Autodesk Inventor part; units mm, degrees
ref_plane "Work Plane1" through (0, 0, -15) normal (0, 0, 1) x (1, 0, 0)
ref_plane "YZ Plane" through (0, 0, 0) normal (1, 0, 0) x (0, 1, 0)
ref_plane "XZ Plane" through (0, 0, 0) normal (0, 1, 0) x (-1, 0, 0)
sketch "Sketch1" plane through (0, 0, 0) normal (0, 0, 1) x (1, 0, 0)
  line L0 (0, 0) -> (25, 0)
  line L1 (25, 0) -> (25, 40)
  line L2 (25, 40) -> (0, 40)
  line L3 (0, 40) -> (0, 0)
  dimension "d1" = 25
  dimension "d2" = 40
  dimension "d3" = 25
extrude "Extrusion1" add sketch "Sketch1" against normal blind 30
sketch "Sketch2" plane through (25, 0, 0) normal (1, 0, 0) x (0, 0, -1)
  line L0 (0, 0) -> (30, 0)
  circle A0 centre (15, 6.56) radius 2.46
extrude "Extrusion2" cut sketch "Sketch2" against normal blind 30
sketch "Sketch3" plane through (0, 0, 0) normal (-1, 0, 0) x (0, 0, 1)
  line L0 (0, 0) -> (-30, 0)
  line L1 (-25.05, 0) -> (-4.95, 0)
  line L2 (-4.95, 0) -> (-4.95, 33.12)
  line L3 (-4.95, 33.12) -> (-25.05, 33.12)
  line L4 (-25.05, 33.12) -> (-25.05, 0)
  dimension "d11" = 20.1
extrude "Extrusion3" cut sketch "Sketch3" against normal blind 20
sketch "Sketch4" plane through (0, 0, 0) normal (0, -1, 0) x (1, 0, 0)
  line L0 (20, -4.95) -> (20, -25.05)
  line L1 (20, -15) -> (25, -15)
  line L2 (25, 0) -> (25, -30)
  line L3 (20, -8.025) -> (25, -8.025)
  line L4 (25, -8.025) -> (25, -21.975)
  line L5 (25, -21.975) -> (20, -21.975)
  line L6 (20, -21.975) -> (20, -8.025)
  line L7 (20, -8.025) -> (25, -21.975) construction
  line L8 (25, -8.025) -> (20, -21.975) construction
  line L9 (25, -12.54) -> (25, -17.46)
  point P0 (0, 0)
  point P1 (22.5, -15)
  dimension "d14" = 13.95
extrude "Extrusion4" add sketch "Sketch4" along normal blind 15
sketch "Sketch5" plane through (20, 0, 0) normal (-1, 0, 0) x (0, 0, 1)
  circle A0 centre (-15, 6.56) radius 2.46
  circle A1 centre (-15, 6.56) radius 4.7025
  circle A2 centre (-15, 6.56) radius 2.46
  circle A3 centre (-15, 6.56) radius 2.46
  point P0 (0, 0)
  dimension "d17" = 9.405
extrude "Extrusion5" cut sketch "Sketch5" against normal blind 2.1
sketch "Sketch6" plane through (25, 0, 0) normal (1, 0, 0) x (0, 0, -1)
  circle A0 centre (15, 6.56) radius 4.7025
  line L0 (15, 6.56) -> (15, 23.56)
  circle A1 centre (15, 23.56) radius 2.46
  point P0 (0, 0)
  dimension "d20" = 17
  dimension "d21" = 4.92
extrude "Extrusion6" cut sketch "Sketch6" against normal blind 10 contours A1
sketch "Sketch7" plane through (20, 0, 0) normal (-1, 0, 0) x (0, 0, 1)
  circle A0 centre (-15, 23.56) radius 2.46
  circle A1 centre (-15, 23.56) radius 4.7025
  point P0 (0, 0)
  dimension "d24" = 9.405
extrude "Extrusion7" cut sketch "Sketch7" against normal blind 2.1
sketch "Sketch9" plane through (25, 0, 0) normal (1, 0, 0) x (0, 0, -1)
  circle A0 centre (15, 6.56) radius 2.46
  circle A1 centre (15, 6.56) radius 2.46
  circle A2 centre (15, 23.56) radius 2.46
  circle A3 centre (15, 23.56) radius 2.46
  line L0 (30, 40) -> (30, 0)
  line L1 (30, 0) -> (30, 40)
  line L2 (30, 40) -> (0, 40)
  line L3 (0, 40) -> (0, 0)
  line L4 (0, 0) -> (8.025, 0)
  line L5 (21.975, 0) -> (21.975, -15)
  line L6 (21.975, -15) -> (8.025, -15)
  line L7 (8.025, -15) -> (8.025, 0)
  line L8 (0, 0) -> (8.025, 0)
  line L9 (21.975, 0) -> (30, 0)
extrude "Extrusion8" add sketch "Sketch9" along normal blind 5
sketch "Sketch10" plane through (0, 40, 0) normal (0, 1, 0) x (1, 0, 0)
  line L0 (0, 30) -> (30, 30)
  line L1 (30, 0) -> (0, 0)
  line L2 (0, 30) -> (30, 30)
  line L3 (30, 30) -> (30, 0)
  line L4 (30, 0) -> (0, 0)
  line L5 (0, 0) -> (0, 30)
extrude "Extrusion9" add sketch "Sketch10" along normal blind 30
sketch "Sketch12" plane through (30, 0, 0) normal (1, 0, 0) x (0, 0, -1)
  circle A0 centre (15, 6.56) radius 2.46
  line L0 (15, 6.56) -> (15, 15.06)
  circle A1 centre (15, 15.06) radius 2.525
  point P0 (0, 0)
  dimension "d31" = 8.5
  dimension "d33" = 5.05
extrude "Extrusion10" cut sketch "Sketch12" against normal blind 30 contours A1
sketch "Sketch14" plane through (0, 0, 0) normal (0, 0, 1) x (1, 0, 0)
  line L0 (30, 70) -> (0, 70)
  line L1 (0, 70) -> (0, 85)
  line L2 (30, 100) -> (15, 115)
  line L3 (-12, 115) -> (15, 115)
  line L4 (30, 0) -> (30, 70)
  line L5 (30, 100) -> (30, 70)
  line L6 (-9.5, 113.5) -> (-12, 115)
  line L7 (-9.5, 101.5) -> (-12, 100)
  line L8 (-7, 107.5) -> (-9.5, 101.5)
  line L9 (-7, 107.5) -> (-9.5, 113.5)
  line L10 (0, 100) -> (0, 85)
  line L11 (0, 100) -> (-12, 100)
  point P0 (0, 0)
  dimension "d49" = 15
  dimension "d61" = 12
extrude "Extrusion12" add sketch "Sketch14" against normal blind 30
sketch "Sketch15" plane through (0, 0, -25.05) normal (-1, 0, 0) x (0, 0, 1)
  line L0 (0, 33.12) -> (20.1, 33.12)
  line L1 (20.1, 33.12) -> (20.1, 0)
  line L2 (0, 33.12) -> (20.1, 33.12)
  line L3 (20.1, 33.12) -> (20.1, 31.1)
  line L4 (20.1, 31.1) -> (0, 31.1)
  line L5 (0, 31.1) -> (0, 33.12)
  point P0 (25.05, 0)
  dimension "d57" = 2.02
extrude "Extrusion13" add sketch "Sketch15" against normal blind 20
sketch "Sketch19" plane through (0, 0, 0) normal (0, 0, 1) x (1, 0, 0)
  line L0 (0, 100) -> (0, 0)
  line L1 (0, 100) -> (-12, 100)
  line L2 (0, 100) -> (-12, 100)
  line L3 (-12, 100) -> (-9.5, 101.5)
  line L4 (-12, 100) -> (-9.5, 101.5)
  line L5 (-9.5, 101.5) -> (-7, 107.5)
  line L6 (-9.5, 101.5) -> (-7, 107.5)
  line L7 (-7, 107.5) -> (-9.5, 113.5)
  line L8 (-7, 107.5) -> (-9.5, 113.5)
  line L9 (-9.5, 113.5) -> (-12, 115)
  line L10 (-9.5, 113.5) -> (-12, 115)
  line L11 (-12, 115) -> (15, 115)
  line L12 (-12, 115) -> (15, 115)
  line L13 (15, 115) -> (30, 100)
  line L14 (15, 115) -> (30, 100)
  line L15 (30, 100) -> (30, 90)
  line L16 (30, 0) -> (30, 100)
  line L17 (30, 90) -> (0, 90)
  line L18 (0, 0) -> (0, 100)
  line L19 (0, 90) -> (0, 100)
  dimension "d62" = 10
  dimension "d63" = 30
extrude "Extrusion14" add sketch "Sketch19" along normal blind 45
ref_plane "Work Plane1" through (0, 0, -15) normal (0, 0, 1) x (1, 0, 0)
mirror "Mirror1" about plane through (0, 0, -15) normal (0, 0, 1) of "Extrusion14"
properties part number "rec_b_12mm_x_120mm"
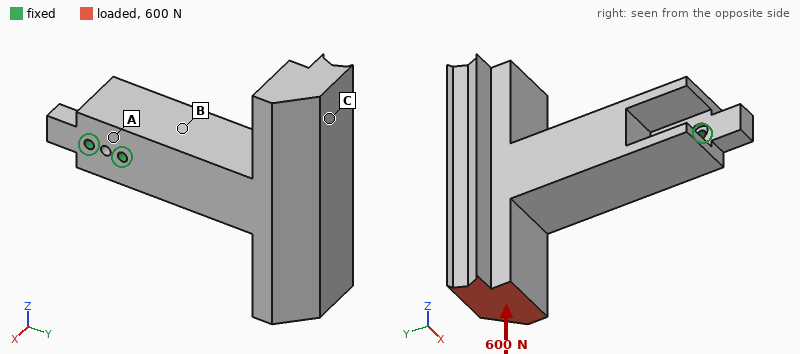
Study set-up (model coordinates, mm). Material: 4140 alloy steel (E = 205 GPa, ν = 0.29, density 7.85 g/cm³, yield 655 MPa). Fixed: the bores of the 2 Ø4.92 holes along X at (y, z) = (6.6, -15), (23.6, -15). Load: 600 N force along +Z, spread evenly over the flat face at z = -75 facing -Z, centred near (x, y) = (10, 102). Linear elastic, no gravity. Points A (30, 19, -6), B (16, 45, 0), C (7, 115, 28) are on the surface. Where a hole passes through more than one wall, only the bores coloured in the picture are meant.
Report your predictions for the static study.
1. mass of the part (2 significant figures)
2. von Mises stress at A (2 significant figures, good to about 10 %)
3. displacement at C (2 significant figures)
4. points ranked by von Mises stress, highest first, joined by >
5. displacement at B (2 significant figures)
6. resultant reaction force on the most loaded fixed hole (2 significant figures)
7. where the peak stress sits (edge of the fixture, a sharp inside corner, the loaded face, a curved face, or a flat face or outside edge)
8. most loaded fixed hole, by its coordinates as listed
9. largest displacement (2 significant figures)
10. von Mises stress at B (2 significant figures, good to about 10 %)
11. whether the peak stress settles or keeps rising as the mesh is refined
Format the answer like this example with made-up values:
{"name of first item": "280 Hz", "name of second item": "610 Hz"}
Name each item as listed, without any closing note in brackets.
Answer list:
{"mass of the part": "1.3 kg", "von Mises stress at A": "16 MPa", "displacement at C": "33 µm", "points ranked by von Mises stress, highest first, joined by >": "A > B > C", "displacement at B": "7.5 µm", "resultant reaction force on the most loaded fixed hole": "2.6 kN", "where the peak stress sits": "edge of the fixture", "most loaded fixed hole, by its coordinates as listed": "(23.6, -15)", "largest displacement": "38 µm", "von Mises stress at B": "8.3 MPa", "whether the peak stress settles or keeps rising as the mesh is refined": "keeps rising"}
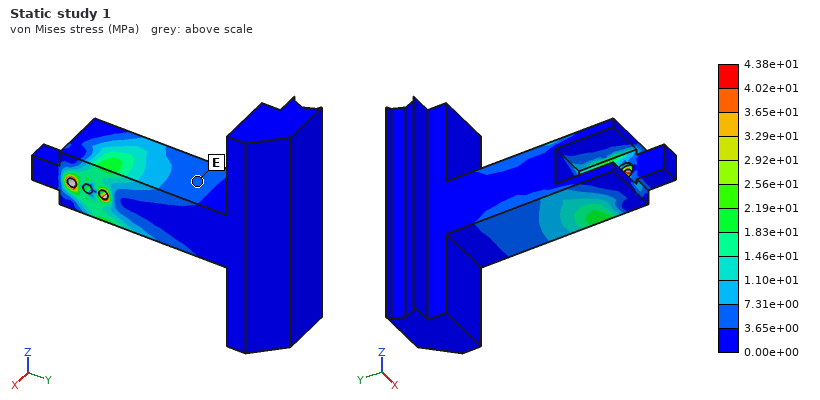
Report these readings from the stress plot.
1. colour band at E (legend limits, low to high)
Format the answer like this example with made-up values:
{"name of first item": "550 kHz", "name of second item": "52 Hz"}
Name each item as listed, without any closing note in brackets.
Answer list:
{"colour band at E": "3.65e+00 to 7.31e+00 MPa"}
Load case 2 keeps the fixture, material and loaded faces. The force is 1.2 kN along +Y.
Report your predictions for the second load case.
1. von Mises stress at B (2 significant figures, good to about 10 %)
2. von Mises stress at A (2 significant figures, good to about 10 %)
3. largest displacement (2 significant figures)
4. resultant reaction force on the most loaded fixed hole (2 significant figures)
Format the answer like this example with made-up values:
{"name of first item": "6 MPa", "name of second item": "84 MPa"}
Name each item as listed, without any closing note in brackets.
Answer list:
{"von Mises stress at B": "16 MPa", "von Mises stress at A": "26 MPa", "largest displacement": "82 µm", "resultant reaction force on the most loaded fixed hole": "3.3 kN"}
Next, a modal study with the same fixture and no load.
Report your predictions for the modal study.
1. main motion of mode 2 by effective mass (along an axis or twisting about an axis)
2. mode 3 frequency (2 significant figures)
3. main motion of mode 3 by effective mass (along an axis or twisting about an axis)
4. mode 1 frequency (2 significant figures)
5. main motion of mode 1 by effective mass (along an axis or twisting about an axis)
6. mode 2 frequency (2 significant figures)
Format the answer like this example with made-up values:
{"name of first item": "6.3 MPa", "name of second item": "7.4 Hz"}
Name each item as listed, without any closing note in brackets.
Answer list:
{"main motion of mode 2 by effective mass": "along Z", "mode 3 frequency": "1100 Hz", "main motion of mode 3 by effective mass": "twisting about Y", "mode 1 frequency": "720 Hz", "main motion of mode 1 by effective mass": "along X", "mode 2 frequency": "770 Hz"}
